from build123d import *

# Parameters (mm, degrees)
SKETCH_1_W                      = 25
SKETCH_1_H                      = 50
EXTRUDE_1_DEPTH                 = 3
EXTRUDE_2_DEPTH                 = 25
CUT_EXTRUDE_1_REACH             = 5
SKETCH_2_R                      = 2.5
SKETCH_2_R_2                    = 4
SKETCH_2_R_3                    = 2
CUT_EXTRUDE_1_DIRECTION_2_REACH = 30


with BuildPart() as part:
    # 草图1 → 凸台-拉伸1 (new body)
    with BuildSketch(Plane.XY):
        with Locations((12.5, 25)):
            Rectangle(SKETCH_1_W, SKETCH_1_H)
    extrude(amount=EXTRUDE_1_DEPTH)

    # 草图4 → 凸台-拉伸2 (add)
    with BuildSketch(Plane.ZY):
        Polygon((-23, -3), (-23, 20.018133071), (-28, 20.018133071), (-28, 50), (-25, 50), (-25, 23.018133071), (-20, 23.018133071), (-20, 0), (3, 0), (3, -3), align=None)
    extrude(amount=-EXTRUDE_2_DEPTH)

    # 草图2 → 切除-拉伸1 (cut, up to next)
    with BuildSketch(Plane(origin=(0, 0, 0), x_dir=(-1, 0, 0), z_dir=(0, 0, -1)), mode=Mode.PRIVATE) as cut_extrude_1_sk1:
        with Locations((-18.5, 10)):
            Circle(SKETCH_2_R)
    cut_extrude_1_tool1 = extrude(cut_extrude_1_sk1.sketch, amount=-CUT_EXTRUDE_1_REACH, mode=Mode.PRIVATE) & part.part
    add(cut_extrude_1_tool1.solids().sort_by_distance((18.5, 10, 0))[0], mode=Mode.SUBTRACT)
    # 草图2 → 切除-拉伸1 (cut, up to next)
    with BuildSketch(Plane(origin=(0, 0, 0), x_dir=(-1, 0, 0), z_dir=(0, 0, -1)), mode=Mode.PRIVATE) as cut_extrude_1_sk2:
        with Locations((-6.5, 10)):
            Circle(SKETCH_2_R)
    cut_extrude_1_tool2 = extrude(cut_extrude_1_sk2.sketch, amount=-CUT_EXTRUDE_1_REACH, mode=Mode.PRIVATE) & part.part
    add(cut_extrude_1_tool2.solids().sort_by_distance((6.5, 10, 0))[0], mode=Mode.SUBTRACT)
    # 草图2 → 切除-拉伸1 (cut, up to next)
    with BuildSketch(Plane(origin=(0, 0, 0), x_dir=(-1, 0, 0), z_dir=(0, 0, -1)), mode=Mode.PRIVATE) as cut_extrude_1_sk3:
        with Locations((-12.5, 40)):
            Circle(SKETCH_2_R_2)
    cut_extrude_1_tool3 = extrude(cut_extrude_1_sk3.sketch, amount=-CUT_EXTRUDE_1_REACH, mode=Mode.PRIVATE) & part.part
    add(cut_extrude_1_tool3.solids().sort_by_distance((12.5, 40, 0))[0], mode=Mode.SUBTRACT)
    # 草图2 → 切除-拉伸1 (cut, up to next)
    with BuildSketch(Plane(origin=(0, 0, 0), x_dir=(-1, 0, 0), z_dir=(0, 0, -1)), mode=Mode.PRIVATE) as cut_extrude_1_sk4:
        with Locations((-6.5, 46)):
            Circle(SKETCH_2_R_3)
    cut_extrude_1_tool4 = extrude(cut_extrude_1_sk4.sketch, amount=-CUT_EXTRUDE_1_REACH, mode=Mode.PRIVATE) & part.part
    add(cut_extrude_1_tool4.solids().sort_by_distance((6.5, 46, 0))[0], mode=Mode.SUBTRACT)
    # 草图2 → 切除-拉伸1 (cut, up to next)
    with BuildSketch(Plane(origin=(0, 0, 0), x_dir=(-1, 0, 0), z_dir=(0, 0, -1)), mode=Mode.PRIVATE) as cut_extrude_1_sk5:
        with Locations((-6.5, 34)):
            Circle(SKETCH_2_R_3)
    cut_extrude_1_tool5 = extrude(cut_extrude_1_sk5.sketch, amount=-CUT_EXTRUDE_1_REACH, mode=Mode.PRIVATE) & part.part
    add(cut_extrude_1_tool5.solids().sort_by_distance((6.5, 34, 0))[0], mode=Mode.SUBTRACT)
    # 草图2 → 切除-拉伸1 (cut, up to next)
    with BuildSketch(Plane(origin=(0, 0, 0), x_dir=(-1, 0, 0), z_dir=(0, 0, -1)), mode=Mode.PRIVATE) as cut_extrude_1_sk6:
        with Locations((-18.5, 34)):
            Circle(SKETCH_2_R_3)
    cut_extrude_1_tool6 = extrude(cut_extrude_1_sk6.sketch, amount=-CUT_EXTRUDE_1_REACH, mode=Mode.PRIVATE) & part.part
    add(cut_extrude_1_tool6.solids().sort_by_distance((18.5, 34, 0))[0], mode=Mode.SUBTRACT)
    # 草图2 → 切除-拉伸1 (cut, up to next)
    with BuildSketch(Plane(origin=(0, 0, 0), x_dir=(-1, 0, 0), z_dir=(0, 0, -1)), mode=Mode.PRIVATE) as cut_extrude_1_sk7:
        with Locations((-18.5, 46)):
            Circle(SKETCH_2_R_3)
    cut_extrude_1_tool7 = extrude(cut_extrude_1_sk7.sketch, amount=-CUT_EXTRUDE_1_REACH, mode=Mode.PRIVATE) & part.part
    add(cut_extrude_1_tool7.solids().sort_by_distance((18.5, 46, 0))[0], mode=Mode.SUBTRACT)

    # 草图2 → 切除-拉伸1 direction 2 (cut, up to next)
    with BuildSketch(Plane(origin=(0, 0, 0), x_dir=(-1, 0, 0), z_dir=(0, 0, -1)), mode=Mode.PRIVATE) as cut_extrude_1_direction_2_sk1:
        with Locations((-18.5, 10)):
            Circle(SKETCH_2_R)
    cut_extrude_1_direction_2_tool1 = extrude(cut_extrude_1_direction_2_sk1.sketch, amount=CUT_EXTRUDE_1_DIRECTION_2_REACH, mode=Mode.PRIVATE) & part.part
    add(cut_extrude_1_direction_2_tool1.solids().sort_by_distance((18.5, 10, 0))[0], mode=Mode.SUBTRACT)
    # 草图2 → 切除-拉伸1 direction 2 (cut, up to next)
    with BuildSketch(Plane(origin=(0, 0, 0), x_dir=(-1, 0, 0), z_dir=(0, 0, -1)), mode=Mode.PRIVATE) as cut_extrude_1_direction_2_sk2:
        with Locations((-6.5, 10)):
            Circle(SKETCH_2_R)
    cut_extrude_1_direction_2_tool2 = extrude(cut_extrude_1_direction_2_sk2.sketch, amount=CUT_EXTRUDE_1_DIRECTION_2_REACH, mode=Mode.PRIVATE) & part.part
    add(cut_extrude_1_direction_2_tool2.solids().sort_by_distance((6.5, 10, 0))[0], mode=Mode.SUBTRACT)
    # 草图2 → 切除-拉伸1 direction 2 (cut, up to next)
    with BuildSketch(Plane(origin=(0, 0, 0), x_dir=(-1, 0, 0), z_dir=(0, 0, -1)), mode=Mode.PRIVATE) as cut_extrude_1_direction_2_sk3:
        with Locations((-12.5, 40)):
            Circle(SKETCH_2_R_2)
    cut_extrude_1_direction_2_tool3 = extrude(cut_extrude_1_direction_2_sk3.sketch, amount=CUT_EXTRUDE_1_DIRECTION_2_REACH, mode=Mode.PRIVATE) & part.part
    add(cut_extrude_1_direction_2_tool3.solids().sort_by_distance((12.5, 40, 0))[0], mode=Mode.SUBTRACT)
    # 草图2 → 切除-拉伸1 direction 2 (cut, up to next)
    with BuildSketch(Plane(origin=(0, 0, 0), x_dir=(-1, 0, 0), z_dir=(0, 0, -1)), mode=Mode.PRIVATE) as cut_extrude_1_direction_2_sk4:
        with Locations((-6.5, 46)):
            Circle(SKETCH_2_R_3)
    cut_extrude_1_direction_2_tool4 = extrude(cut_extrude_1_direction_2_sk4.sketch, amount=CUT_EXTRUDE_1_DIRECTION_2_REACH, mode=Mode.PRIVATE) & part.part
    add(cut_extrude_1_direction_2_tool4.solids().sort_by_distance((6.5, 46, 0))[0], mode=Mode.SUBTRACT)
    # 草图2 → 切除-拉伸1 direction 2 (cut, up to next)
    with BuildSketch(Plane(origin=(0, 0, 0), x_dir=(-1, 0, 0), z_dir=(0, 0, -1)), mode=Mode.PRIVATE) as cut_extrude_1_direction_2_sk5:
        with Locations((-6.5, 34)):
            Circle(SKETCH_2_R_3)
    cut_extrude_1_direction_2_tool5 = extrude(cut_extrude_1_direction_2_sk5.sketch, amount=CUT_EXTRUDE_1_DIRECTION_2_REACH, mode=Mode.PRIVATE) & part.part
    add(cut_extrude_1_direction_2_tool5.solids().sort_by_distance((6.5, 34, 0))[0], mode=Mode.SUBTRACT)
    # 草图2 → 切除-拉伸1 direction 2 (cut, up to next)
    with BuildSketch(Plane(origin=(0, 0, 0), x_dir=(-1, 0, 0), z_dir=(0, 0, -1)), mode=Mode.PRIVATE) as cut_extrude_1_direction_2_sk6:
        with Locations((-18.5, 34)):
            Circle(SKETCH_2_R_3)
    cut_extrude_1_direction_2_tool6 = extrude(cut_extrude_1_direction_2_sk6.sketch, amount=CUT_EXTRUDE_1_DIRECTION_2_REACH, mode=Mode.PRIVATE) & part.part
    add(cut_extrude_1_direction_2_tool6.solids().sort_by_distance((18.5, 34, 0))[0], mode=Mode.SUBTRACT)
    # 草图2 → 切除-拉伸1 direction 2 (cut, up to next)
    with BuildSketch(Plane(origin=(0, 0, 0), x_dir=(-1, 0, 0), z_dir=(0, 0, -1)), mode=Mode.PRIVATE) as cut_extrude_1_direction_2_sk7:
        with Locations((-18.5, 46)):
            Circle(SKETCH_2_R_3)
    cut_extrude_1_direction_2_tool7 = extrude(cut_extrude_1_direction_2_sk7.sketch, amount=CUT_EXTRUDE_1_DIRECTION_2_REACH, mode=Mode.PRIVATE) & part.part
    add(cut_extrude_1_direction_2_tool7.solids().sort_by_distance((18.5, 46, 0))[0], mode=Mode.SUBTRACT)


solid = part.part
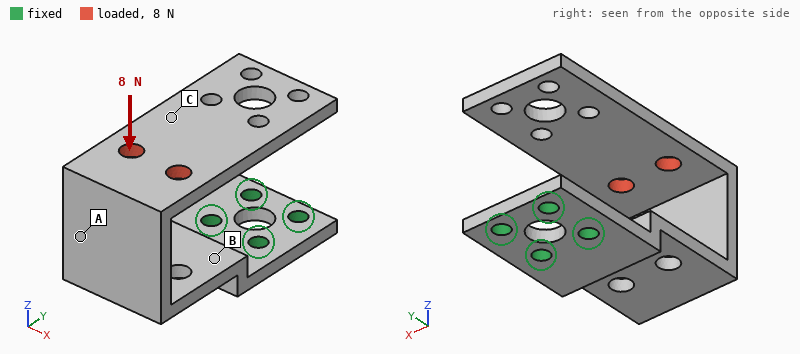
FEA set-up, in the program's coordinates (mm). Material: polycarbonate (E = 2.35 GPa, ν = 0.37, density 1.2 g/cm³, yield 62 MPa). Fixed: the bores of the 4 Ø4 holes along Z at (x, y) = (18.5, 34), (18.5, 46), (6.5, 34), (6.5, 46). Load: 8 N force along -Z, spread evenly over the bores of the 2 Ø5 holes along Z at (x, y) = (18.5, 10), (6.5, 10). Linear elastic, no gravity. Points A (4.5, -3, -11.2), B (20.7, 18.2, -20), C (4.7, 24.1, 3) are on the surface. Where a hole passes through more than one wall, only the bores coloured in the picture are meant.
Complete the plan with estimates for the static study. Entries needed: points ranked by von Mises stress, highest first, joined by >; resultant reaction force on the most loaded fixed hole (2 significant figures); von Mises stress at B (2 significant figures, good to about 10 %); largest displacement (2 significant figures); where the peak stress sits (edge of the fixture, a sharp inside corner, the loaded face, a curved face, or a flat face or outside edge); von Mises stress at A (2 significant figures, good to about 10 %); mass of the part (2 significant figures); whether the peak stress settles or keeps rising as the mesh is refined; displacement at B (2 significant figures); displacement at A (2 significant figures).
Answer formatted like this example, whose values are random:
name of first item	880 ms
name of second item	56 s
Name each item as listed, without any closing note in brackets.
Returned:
points ranked by von Mises stress, highest first, joined by >	A > B > C
resultant reaction force on the most loaded fixed hole	4.6 N
von Mises stress at B	1.6 MPa
largest displacement	0.67 mm
where the peak stress sits	edge of the fixture
von Mises stress at A	2.2 MPa
mass of the part	11 g
whether the peak stress settles or keeps rising as the mesh is refined	keeps rising
displacement at B	0.15 mm
displacement at A	0.48 mm
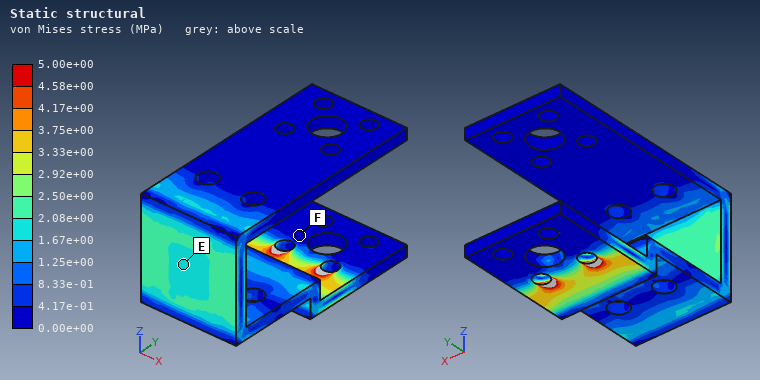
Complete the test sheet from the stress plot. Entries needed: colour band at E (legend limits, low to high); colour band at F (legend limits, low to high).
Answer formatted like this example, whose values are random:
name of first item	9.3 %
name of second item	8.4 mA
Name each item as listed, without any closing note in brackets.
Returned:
colour band at E	1.67e+00 to 2.08e+00 MPa
colour band at F	0.00e+00 to 4.17e-01 MPa
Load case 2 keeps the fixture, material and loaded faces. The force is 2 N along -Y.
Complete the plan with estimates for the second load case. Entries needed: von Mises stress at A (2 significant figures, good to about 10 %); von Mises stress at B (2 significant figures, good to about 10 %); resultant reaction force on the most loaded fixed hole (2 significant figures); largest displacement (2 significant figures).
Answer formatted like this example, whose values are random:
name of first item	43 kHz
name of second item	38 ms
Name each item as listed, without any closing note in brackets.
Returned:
von Mises stress at A	0.64 MPa
von Mises stress at B	1.1 MPa
resultant reaction force on the most loaded fixed hole	1.1 N
largest displacement	0.78 mm
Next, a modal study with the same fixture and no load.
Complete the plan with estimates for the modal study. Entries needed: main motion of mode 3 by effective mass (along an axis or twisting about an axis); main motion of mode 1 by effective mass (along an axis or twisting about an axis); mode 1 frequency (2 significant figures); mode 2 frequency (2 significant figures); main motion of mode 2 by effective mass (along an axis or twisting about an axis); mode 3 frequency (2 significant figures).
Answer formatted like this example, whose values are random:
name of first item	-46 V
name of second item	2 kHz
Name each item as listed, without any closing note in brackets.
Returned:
main motion of mode 3 by effective mass	along Z
main motion of mode 1 by effective mass	along Y
mode 1 frequency	120 Hz
mode 2 frequency	180 Hz
main motion of mode 2 by effective mass	along X
mode 3 frequency	200 Hz
